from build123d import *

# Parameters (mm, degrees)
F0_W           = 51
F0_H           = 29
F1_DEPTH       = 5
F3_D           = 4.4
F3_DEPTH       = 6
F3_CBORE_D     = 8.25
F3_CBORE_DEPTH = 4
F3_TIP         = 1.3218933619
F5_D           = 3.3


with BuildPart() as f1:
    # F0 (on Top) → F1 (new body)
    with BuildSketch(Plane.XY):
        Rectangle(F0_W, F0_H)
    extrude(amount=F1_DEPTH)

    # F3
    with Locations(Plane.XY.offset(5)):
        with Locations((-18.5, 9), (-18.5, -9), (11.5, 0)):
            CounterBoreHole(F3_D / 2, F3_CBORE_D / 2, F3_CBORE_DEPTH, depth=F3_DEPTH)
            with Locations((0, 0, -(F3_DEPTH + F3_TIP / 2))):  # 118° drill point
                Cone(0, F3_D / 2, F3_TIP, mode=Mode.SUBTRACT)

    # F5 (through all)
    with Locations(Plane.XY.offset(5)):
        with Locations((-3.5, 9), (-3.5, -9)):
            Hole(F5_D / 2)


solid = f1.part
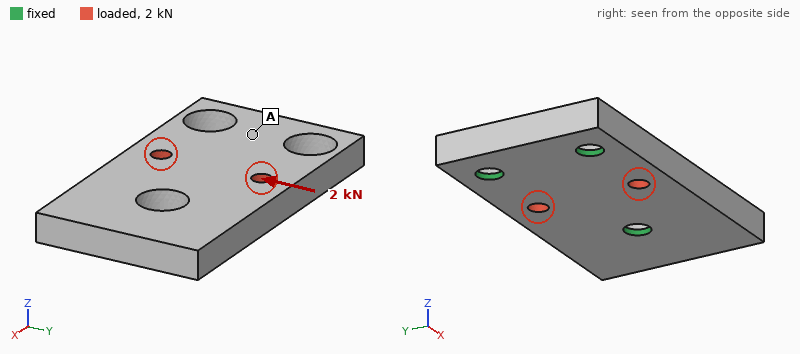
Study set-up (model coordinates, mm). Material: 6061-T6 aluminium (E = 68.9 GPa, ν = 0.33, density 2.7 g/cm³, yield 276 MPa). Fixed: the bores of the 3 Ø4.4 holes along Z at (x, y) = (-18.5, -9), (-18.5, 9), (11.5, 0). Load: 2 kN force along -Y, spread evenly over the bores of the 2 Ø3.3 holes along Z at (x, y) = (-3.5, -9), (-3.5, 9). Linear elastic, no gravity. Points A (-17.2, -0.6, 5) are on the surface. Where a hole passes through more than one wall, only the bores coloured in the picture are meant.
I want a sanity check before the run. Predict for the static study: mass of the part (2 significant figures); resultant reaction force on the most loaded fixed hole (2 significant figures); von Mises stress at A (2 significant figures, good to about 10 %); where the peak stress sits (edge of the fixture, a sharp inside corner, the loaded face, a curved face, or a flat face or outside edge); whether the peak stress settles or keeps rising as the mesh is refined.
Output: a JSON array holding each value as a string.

["18 g", "790 N", "20 MPa", "edge of the fixture", "keeps rising"]
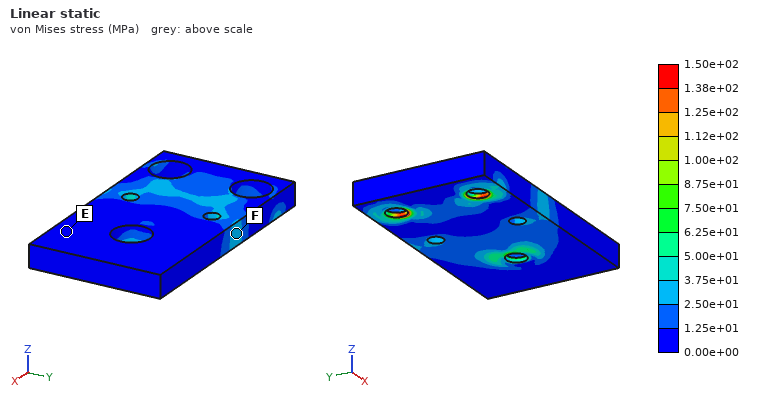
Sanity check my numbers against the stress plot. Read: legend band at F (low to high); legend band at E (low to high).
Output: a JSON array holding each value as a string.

["2.50e+01 to 3.75e+01 MPa", "0.00e+00 to 1.25e+01 MPa"]
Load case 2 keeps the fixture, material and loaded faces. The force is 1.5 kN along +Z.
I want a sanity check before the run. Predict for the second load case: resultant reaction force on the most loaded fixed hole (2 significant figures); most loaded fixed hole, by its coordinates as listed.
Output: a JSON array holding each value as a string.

["1.3 kN", "(11.5, 0)"]
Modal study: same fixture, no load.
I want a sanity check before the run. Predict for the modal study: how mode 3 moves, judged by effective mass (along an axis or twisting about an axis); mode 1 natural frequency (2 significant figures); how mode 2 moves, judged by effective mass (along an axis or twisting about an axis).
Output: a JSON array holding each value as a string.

["along Z", "6900 Hz", "along Z"]
